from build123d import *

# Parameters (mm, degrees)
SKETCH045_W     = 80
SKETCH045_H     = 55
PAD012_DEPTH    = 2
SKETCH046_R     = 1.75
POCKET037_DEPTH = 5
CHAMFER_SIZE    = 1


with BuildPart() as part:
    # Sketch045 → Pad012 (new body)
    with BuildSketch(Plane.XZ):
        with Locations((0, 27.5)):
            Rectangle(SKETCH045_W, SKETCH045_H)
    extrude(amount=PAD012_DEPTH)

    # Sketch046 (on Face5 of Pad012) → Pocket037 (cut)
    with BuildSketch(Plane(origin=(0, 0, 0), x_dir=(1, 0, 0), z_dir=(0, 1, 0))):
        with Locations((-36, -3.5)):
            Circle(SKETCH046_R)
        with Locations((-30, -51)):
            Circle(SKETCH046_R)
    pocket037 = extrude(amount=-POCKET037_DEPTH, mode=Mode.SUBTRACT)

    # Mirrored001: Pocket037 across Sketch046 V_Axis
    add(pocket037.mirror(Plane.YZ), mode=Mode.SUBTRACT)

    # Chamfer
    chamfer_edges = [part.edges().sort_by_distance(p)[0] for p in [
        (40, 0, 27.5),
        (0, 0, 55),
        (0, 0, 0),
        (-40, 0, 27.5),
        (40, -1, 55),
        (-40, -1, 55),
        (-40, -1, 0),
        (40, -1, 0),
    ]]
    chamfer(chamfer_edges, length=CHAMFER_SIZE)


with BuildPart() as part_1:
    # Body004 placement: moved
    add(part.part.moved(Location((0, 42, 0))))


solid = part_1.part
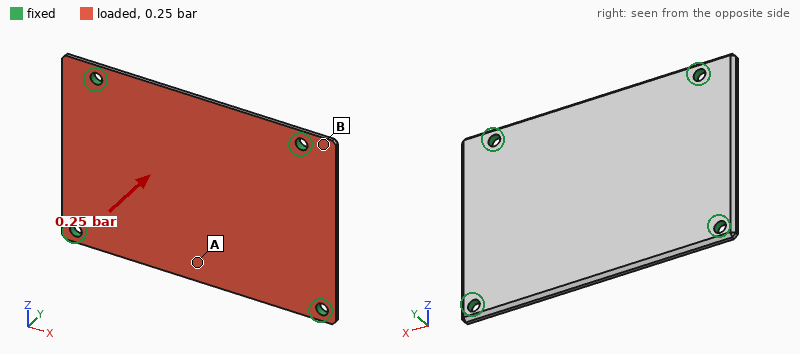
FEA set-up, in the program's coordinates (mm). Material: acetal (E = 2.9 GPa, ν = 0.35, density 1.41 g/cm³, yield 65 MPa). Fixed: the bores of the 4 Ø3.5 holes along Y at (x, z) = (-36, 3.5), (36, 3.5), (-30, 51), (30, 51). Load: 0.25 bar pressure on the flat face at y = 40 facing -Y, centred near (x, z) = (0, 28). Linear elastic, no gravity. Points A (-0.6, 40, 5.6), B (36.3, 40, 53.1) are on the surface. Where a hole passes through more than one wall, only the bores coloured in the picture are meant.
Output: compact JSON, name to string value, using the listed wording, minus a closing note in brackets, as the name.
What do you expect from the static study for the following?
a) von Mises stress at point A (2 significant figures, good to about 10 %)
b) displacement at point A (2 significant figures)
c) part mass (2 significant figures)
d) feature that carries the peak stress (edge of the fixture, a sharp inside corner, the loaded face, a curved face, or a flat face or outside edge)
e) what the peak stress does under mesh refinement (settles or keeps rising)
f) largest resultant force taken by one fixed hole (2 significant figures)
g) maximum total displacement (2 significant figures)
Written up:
{"von Mises stress at point A": "8.9 MPa", "displacement at point A": "1.1 mm", "part mass": "12 g", "feature that carries the peak stress": "edge of the fixture", "what the peak stress does under mesh refinement": "keeps rising", "largest resultant force taken by one fixed hole": "29 N", "maximum total displacement": "1.2 mm"}
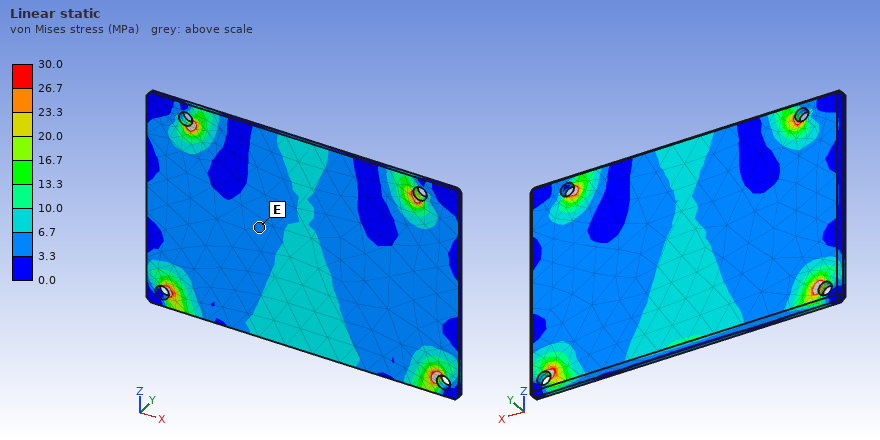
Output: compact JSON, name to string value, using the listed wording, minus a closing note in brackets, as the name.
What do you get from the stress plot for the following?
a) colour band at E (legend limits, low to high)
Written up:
{"colour band at E": "3.3 to 6.7 MPa"}
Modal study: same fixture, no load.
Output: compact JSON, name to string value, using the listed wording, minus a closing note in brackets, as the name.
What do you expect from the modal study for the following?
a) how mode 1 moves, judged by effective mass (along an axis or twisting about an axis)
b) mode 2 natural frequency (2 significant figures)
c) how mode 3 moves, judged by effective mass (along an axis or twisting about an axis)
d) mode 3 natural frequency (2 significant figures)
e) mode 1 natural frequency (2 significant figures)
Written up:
{"how mode 1 moves, judged by effective mass": "along Y", "mode 2 natural frequency": "920 Hz", "how mode 3 moves, judged by effective mass": "twisting about Z", "mode 3 natural frequency": "1200 Hz", "mode 1 natural frequency": "540 Hz"}
